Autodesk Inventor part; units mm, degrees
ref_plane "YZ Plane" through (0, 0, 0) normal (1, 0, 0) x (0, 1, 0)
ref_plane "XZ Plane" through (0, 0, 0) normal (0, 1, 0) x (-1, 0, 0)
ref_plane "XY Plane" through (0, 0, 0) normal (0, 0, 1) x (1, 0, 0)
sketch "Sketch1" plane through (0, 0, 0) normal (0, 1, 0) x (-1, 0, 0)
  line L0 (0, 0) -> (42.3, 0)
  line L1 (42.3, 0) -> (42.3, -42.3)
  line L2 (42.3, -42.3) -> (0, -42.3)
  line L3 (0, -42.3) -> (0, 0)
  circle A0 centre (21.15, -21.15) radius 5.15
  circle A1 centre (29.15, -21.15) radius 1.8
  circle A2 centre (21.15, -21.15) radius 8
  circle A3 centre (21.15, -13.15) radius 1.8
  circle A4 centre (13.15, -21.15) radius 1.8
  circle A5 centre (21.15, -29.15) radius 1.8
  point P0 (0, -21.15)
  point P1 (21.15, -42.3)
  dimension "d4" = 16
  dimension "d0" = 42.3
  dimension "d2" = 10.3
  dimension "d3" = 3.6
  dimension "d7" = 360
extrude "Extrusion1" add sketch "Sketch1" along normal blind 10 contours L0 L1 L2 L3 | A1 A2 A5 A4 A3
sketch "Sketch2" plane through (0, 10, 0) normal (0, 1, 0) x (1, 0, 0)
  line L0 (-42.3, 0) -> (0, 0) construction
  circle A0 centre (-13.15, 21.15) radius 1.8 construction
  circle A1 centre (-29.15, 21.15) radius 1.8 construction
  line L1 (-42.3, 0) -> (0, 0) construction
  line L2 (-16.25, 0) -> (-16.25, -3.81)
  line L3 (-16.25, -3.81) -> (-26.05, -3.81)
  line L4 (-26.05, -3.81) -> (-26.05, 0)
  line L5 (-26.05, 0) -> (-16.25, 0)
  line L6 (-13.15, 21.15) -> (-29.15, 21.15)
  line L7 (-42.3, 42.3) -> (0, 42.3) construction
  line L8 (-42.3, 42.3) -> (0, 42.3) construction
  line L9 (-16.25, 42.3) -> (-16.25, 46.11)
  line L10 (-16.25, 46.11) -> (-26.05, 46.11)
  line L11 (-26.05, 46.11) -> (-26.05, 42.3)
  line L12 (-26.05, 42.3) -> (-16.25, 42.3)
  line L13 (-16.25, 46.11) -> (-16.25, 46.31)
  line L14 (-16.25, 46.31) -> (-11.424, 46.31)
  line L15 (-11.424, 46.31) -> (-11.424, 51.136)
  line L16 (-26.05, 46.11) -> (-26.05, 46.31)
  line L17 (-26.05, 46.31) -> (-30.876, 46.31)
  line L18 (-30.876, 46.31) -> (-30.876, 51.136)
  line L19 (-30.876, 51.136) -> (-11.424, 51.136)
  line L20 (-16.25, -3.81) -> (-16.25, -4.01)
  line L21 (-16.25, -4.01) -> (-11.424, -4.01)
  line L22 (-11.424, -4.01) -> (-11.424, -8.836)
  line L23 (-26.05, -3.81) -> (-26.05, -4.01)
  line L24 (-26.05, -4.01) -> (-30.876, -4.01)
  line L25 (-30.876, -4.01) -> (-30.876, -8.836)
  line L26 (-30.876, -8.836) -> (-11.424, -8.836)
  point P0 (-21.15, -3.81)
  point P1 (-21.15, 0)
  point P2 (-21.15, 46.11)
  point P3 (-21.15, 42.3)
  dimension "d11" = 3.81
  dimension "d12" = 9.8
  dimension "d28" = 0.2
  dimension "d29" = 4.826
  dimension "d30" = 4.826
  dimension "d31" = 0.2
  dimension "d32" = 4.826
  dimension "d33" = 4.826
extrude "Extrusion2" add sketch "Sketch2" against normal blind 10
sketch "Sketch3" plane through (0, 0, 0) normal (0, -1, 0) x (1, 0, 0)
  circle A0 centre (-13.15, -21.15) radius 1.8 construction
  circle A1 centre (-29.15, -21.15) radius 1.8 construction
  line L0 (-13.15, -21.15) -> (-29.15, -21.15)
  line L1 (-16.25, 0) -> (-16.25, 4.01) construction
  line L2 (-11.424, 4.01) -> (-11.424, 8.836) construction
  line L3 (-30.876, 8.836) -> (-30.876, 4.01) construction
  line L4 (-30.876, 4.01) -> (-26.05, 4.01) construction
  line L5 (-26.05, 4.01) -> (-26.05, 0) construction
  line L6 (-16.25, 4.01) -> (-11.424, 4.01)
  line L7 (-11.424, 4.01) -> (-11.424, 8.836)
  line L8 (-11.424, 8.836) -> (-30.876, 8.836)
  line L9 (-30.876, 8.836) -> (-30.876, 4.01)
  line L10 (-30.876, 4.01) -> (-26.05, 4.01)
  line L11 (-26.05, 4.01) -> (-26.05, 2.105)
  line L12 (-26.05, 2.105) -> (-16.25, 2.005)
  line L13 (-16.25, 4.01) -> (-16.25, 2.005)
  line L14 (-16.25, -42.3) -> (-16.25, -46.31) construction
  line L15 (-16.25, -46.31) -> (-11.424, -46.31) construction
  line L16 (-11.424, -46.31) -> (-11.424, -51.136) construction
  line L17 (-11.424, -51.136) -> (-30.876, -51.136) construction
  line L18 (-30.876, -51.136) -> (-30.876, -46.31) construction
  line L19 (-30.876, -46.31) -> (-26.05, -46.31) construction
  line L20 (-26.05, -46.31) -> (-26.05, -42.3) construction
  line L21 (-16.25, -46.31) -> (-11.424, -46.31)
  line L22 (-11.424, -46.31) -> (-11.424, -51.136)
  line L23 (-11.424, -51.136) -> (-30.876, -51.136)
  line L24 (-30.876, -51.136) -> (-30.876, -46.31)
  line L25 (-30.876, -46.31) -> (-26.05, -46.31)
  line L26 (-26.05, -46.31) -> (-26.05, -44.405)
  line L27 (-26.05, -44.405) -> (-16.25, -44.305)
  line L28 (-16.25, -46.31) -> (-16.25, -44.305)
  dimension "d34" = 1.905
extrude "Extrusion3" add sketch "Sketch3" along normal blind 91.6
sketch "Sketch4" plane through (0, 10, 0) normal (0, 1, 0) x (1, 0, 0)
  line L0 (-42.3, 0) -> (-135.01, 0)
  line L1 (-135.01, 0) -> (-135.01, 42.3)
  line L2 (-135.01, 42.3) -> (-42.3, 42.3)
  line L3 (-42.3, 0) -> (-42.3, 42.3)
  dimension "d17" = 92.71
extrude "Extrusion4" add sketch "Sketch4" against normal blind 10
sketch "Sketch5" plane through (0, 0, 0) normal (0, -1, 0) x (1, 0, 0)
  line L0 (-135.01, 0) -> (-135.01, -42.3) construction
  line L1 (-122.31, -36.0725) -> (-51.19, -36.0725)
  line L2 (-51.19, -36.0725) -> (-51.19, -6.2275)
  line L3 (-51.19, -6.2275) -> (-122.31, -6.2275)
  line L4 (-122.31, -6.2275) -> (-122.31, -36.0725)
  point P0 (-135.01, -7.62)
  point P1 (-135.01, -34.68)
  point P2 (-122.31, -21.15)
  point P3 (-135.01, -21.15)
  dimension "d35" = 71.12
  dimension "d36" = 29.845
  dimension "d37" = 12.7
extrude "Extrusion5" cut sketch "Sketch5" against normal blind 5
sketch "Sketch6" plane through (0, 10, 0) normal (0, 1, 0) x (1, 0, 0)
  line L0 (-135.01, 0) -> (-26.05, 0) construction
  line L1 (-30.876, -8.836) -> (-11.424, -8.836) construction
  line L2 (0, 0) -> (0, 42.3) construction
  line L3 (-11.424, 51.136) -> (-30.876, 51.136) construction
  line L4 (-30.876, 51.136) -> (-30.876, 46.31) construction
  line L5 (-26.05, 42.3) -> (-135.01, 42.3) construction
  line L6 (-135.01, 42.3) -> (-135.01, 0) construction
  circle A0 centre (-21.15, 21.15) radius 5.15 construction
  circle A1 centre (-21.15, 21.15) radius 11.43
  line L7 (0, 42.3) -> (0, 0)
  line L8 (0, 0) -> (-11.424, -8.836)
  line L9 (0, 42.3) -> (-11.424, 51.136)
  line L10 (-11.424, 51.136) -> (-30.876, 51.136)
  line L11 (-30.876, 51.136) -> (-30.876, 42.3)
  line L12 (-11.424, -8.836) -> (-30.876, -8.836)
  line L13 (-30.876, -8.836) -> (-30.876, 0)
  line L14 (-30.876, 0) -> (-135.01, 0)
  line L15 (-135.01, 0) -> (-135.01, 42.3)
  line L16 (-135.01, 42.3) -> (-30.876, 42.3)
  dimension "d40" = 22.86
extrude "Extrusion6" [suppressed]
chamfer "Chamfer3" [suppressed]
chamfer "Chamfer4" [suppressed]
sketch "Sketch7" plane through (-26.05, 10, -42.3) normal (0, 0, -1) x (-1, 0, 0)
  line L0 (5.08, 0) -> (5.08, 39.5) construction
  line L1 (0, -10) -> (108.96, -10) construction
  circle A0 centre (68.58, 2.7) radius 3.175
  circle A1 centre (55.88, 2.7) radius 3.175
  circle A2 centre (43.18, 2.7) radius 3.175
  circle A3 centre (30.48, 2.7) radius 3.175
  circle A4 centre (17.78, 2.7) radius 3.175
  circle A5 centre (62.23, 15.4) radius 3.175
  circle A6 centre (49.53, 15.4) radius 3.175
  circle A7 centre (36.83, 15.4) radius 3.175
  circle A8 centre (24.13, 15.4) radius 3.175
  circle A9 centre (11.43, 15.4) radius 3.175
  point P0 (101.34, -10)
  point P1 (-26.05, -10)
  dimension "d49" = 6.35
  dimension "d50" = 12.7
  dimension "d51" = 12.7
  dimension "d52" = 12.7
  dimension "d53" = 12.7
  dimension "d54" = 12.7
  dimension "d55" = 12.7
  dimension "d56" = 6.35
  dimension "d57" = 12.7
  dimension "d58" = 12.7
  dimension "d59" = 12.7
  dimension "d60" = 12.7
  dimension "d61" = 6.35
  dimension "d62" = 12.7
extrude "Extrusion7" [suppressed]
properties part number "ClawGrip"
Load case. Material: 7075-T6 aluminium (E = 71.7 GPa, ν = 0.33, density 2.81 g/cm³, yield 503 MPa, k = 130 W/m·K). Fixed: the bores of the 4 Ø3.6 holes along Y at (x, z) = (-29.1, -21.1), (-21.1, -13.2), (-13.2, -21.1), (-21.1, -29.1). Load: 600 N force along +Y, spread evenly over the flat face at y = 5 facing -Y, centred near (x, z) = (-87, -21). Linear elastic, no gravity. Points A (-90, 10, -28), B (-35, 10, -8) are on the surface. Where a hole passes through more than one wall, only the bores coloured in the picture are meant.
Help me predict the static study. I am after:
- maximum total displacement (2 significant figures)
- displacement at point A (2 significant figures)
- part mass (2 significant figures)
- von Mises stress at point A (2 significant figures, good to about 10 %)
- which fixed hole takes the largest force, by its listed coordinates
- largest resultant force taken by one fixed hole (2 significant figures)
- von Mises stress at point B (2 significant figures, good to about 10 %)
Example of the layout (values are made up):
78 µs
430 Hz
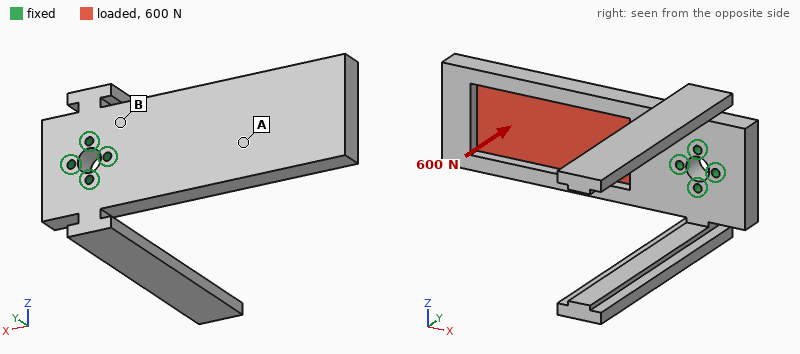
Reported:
0.58 mm
0.26 mm
190 g
11 MPa
(-29.1, -21.1)
1.6 kN
36 MPa
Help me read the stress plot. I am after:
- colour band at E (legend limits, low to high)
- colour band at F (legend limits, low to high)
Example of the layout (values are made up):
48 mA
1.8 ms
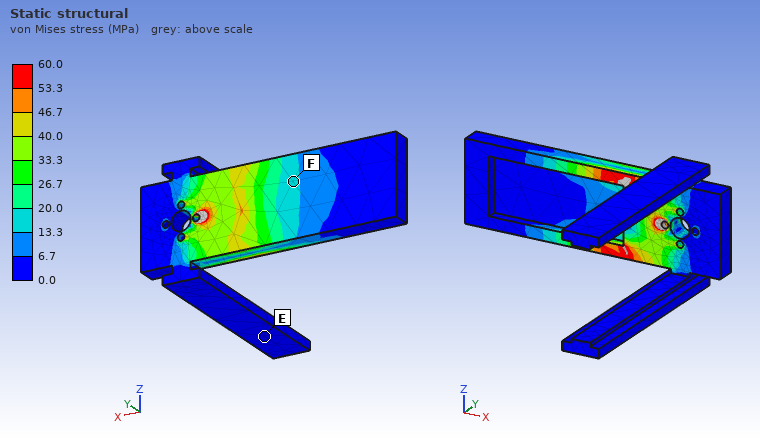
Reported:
0.0 to 6.7 MPa
13.3 to 20.0 MPa
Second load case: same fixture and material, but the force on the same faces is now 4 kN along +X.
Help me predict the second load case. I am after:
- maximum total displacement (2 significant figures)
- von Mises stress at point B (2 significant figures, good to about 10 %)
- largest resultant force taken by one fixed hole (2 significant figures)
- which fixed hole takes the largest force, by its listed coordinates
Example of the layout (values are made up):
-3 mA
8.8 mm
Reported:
0.12 mm
8.4 MPa
1.5 kN
(-29.1, -21.1)
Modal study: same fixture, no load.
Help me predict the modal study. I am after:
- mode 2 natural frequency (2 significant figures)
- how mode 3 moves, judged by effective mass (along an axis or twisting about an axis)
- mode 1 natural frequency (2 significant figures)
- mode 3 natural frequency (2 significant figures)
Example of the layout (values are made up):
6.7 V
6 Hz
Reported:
510 Hz
along Y
510 Hz
640 Hz
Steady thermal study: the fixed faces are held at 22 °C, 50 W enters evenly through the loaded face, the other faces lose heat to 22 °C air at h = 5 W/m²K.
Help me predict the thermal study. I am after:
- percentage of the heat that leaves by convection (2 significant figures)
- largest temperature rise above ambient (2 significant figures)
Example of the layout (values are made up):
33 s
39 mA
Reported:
5.4 %
72 K
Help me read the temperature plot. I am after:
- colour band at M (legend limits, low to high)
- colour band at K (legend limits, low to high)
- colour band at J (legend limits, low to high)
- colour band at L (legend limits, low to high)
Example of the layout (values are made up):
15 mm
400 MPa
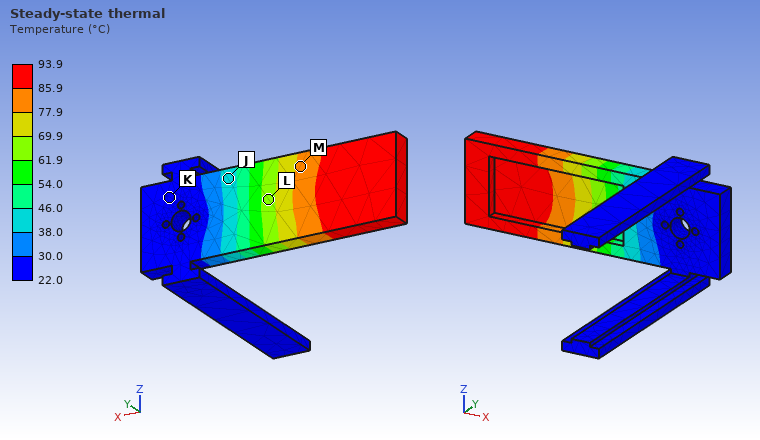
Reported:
77.9 to 85.9 °C
22.0 to 30.0 °C
38.0 to 46.0 °C
61.9 to 69.9 °C
